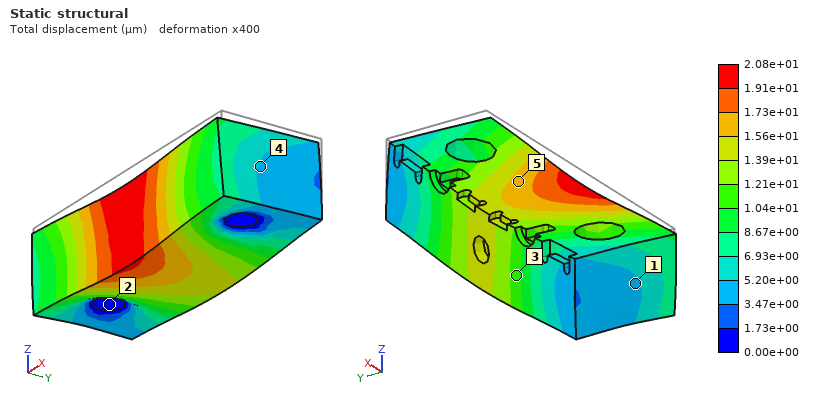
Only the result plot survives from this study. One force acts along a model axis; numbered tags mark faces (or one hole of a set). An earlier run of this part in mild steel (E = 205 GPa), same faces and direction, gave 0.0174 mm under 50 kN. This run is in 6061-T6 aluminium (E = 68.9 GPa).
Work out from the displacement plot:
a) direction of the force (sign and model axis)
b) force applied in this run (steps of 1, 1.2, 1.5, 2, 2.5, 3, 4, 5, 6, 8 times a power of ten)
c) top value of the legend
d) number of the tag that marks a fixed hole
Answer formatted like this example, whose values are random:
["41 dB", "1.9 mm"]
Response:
["-Z", "20 kN", "2.08e+01 µm", "2"]
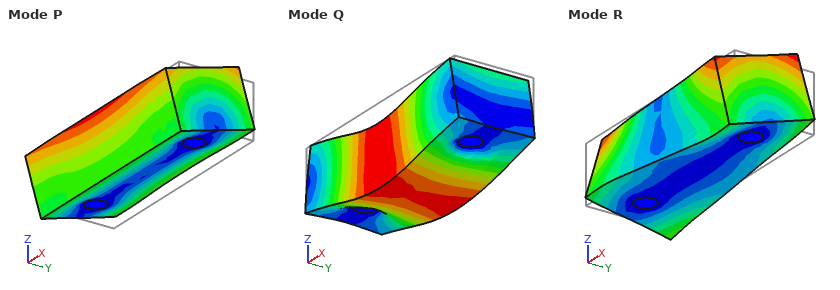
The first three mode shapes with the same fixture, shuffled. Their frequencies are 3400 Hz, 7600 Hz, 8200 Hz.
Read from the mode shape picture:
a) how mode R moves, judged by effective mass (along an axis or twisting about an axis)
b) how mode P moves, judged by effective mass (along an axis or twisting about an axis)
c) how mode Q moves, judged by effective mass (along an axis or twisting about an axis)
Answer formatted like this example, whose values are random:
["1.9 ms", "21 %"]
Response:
["twisting about Z", "along Y", "along Z"]
